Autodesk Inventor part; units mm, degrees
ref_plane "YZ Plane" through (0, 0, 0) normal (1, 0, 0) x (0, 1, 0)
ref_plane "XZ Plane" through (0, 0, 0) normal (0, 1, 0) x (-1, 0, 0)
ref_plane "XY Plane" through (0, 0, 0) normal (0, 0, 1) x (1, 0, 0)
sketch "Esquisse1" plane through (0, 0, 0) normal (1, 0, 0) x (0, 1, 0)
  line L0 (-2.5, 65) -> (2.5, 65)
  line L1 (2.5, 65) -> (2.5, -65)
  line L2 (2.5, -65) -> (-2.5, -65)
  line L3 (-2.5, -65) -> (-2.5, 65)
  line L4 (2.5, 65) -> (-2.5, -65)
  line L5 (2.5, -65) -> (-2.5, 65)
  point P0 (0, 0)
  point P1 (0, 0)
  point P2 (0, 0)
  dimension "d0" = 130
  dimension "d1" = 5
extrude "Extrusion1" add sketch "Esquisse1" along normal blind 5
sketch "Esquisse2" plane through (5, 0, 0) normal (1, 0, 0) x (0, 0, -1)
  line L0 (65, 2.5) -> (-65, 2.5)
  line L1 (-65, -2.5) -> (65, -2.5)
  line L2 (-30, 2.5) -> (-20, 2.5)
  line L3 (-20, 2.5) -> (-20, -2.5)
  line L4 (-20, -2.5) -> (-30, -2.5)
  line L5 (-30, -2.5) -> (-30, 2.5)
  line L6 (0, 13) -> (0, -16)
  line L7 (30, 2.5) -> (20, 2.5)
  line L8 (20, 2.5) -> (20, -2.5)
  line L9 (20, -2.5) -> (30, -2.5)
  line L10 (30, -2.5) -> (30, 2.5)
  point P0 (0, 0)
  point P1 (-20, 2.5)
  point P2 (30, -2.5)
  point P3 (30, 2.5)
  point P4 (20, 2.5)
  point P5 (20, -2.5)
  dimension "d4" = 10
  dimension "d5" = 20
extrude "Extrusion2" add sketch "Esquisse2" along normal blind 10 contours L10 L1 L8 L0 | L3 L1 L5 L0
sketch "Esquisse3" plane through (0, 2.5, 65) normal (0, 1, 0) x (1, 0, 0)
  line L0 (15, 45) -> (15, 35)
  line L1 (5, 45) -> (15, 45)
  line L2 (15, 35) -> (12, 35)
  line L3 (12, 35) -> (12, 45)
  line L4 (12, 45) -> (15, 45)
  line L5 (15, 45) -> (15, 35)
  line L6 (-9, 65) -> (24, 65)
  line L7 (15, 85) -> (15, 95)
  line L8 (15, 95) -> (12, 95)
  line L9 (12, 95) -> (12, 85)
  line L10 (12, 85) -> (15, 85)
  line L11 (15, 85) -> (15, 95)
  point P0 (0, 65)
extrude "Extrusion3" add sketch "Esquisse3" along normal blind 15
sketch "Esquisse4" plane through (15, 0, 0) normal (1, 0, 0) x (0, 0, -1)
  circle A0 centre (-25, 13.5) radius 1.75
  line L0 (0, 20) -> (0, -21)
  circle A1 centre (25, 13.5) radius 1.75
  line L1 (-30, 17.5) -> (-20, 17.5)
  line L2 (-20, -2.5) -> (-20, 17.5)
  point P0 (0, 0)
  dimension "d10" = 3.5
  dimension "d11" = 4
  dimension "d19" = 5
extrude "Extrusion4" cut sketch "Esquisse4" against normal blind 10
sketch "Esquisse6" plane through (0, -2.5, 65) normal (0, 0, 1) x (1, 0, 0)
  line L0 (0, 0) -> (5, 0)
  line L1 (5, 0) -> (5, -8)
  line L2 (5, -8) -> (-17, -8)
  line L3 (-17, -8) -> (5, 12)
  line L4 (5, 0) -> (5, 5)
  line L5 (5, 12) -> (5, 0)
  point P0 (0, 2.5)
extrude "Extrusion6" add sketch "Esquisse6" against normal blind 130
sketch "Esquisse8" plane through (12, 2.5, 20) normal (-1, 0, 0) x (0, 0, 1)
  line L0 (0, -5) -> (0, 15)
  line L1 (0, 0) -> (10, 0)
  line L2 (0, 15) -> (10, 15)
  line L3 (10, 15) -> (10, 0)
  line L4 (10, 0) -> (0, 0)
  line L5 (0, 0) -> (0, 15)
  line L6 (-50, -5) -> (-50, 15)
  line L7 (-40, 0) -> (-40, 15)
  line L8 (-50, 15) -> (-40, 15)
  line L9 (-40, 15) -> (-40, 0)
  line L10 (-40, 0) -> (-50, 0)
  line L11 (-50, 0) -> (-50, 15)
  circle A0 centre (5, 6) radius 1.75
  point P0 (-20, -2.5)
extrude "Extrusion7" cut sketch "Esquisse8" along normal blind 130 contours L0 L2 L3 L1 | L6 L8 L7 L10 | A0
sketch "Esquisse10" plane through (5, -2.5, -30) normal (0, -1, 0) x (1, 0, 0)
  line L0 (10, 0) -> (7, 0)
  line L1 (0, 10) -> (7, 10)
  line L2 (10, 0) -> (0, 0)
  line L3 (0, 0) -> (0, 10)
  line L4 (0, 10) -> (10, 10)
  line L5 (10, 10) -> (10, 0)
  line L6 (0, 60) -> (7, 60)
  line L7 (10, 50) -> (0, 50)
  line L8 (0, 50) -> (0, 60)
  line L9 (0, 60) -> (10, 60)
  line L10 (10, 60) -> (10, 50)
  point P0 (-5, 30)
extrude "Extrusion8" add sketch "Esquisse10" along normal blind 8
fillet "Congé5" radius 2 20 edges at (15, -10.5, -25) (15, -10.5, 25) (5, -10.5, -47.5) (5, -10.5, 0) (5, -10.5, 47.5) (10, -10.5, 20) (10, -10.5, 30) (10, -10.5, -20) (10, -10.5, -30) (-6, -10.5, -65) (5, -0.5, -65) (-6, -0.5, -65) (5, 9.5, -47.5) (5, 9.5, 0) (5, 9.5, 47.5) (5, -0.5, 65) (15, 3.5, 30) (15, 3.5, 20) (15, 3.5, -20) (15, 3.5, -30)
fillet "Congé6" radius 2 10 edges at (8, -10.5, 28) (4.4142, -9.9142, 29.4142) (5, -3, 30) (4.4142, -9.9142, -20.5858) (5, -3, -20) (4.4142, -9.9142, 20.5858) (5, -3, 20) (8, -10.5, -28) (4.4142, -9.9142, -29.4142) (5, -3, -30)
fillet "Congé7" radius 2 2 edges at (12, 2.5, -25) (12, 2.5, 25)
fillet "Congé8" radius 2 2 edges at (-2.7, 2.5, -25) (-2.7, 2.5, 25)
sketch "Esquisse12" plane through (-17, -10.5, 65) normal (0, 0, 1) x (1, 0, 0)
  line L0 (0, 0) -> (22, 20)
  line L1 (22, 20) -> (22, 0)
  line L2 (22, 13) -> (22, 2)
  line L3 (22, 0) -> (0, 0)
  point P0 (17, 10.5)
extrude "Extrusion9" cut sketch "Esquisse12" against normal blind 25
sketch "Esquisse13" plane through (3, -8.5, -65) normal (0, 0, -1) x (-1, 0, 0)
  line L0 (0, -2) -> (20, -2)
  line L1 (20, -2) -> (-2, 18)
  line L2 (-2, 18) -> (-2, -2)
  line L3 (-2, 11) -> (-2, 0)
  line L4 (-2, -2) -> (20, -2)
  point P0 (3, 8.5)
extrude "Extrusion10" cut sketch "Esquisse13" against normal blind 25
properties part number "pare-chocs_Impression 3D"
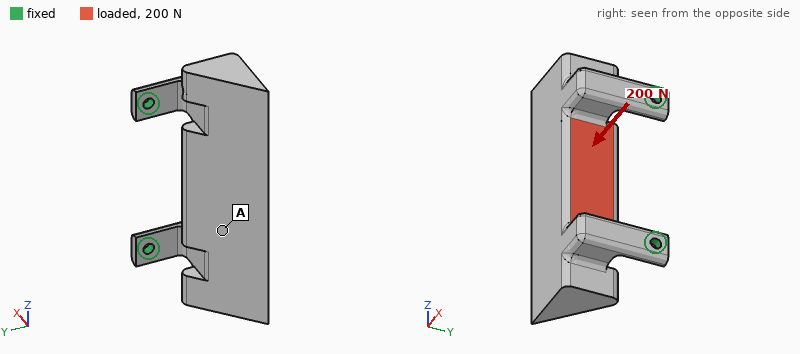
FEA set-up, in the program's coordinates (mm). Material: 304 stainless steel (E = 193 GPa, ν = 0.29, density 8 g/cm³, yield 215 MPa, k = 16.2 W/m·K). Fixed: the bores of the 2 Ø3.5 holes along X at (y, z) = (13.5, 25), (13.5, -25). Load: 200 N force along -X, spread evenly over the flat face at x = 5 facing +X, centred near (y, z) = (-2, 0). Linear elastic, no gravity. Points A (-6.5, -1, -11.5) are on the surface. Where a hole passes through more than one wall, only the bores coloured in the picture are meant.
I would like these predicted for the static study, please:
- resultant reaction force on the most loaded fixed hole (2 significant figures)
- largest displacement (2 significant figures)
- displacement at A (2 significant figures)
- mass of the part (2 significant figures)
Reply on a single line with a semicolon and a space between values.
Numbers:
100 N; 85 µm; 52 µm; 160 g
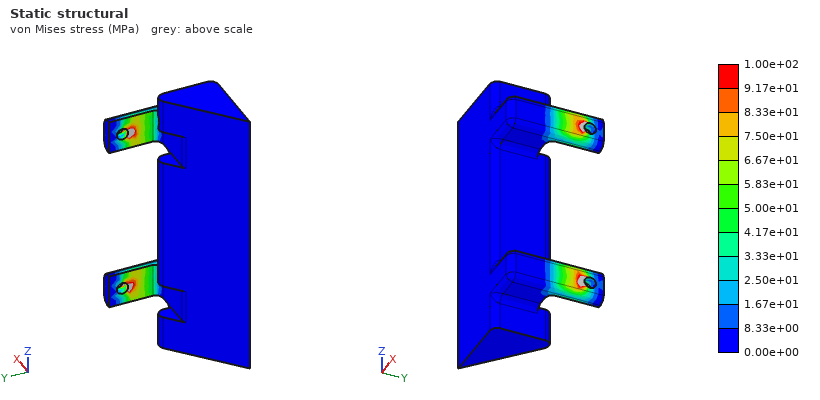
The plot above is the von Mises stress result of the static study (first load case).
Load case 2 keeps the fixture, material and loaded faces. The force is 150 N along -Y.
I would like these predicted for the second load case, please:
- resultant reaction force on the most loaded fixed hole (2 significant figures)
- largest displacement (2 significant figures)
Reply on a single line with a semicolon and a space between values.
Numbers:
75 N; 59 µm
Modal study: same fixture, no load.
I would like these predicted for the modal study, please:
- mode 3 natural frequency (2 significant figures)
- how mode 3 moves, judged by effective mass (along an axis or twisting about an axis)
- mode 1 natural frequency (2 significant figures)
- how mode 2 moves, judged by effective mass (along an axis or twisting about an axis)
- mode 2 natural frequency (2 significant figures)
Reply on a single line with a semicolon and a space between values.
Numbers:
3700 Hz; along Z; 550 Hz; along Z; 2400 Hz
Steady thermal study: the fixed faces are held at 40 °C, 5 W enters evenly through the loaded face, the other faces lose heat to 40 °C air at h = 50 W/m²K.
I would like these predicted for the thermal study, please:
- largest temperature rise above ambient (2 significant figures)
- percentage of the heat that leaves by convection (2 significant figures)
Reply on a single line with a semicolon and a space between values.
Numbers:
24 K; 85 %
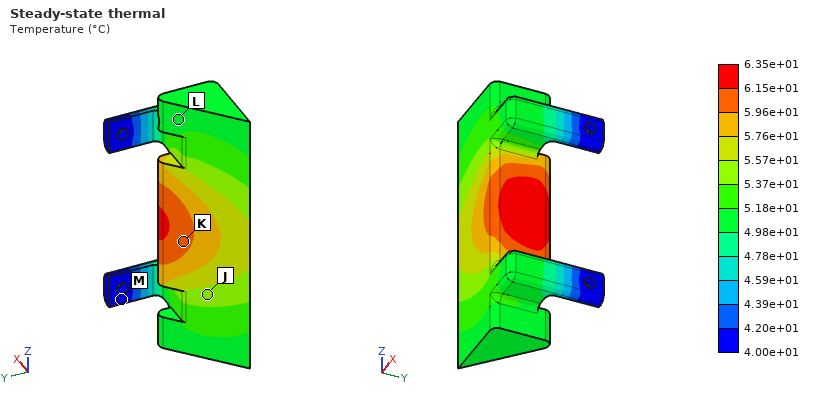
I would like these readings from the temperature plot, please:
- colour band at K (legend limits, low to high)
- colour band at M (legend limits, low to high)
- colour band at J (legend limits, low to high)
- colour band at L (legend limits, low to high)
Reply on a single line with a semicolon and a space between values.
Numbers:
5.96e+01 to 6.15e+01 °C; 4.00e+01 to 4.20e+01 °C; 5.37e+01 to 5.57e+01 °C; 4.98e+01 to 5.18e+01 °C
